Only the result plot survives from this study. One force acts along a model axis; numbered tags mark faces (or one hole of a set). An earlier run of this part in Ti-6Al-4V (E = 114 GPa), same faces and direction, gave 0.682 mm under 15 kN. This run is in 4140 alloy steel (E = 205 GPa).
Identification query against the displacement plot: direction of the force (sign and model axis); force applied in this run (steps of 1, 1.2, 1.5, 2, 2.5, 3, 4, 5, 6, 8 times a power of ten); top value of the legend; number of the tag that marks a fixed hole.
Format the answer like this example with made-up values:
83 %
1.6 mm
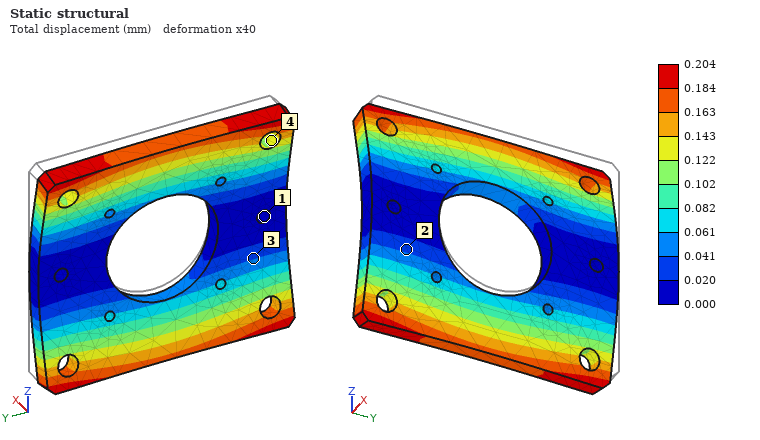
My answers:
-X
8 kN
0.204 mm
1
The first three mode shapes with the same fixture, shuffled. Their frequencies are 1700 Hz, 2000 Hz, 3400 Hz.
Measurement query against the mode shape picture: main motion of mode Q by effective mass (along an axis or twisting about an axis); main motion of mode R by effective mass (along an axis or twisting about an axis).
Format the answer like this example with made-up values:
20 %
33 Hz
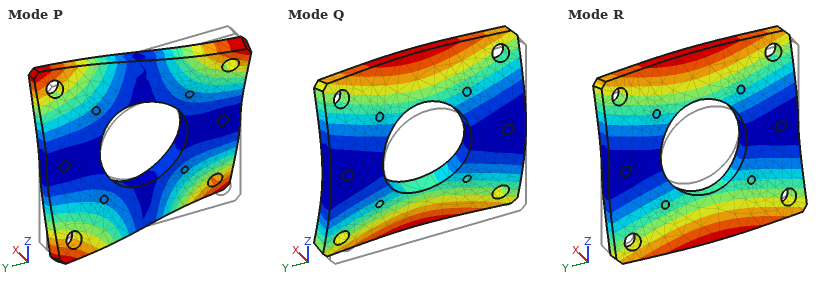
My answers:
along X
twisting about Y
